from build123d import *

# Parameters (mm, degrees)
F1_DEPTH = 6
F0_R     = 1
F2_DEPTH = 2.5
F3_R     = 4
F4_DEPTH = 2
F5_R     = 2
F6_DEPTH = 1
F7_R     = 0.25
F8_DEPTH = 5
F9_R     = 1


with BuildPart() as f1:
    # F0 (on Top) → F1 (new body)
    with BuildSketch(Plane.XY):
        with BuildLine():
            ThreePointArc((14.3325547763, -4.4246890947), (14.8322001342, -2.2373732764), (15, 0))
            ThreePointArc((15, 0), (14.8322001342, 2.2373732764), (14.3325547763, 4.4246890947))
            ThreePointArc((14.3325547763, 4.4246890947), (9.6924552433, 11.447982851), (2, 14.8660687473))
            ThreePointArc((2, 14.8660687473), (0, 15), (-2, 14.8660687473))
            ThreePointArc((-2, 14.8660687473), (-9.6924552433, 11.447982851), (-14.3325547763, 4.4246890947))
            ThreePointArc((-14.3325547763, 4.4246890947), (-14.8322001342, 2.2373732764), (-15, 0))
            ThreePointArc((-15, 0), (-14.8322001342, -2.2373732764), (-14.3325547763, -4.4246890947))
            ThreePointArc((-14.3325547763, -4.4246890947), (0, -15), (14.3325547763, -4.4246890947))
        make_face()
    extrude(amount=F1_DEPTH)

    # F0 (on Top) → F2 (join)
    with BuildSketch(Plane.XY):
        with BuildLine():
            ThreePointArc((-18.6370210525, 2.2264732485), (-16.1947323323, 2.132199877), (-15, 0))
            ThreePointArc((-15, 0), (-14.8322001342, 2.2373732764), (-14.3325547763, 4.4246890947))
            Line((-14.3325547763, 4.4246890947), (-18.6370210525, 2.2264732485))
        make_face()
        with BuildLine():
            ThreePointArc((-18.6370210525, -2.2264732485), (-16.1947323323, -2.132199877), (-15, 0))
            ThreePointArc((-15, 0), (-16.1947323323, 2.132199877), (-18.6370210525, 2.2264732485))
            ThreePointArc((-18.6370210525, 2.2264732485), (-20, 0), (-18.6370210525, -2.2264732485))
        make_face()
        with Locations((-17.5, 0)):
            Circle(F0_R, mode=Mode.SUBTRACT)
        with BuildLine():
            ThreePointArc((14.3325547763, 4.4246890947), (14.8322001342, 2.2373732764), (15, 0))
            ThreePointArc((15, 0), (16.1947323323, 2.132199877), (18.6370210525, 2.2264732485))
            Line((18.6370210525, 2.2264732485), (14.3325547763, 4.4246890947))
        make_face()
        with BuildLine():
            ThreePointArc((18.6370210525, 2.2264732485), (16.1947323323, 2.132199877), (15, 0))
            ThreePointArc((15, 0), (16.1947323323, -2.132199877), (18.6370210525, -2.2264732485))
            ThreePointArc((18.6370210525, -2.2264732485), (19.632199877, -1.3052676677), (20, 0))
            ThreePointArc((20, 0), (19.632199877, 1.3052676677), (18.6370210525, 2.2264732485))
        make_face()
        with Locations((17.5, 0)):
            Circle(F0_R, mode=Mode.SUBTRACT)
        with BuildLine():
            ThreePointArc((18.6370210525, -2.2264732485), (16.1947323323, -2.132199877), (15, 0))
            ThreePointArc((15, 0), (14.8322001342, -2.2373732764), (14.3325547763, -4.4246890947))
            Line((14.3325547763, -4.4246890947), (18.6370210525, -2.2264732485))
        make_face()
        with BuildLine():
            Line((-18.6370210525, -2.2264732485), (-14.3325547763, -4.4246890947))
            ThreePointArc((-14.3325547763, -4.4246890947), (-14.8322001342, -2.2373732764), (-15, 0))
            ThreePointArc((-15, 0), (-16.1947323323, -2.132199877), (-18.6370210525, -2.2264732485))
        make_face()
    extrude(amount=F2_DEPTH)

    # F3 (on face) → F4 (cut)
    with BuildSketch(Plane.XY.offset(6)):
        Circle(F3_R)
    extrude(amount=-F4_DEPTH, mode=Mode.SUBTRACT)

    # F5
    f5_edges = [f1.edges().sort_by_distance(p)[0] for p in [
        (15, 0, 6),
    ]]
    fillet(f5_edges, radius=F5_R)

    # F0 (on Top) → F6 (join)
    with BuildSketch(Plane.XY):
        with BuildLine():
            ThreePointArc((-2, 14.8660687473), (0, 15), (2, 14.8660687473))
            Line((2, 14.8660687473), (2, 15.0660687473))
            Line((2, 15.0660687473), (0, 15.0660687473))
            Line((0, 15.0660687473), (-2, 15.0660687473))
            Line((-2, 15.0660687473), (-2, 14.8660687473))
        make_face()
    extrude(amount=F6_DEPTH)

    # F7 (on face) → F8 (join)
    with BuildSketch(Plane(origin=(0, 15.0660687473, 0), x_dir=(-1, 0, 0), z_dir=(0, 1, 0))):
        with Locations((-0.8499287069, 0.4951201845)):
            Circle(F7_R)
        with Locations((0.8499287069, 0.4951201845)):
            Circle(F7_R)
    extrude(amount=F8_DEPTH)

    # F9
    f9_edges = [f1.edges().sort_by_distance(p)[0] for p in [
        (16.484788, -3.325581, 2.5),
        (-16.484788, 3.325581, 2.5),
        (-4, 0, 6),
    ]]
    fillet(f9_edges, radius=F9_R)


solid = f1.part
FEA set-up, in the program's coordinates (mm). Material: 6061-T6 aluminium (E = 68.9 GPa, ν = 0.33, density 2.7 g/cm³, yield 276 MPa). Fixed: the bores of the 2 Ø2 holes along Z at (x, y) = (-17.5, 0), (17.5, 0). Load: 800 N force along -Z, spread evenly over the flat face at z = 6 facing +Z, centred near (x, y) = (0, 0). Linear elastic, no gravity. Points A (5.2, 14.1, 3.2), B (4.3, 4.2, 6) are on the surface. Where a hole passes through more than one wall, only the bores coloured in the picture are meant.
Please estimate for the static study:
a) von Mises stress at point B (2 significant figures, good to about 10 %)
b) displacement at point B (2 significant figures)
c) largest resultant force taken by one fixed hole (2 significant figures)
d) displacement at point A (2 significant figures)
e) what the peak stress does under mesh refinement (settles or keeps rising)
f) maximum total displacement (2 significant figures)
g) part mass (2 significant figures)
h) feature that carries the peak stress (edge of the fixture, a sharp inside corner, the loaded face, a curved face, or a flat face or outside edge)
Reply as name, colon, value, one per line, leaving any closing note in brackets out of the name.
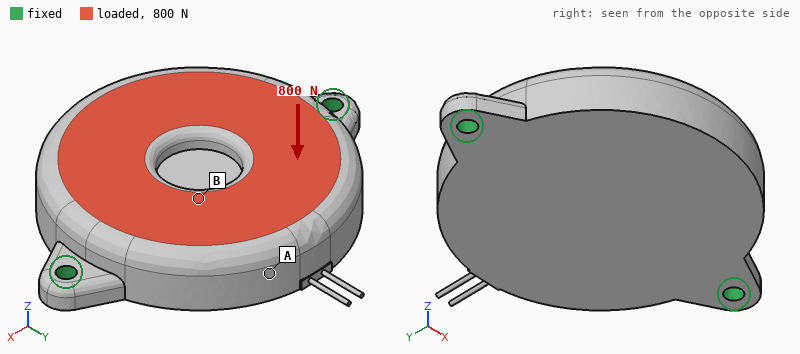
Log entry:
von Mises stress at point B: 29 MPa
displacement at point B: 18 µm
largest resultant force taken by one fixed hole: 540 N
displacement at point A: 23 µm
what the peak stress does under mesh refinement: keeps rising
maximum total displacement: 27 µm
part mass: 11 g
feature that carries the peak stress: edge of the fixture
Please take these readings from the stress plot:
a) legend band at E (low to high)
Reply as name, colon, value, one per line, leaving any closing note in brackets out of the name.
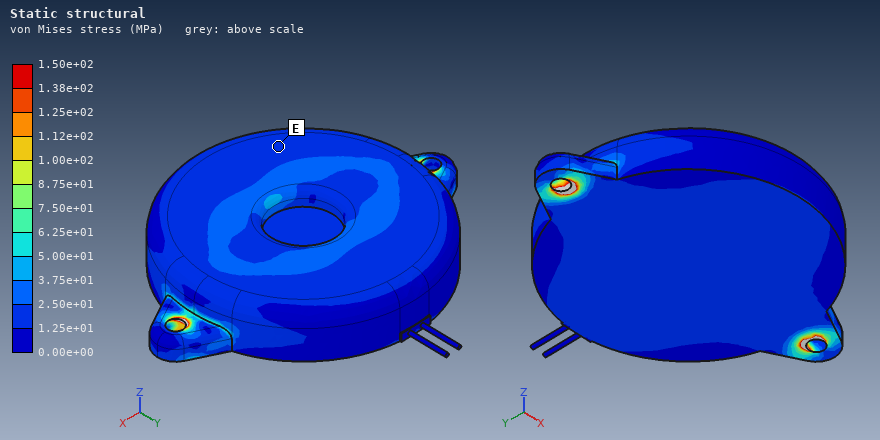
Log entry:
legend band at E: 1.25e+01 to 2.50e+01 MPa
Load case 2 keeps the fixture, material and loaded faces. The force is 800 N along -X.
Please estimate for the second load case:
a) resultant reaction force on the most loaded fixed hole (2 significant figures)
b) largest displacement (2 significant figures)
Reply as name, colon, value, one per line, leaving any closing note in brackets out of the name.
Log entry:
resultant reaction force on the most loaded fixed hole: 420 N
largest displacement: 3.0 µm
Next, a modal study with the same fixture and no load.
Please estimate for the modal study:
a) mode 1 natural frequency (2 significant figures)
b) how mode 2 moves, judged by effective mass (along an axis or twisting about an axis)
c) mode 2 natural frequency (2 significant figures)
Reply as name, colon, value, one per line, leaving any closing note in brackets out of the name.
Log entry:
mode 1 natural frequency: 4400 Hz
how mode 2 moves, judged by effective mass: along Z
mode 2 natural frequency: 10 kHz
